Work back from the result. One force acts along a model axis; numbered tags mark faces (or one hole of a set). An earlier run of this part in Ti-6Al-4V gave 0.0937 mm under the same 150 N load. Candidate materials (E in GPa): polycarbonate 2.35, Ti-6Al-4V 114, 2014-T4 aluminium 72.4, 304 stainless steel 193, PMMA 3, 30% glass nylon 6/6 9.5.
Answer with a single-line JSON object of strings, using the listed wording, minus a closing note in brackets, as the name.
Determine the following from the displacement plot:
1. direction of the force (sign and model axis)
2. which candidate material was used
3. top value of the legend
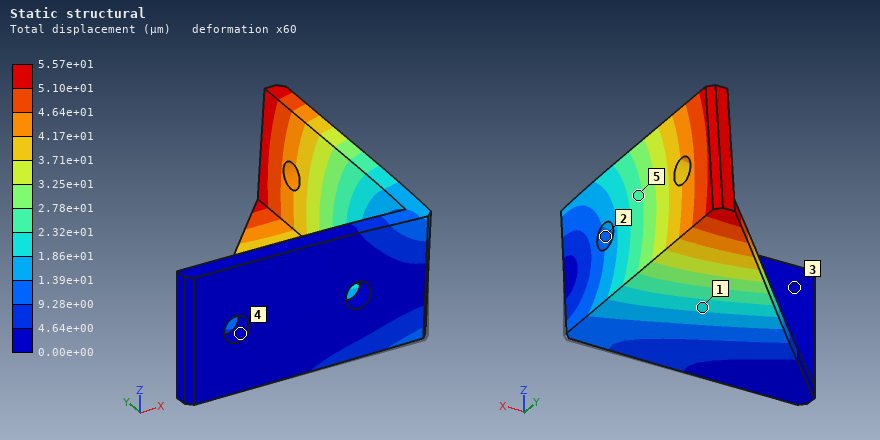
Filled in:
{"direction of the force": "+Z", "which candidate material was used": "304 stainless steel", "top value of the legend": "5.57e+01 µm"}
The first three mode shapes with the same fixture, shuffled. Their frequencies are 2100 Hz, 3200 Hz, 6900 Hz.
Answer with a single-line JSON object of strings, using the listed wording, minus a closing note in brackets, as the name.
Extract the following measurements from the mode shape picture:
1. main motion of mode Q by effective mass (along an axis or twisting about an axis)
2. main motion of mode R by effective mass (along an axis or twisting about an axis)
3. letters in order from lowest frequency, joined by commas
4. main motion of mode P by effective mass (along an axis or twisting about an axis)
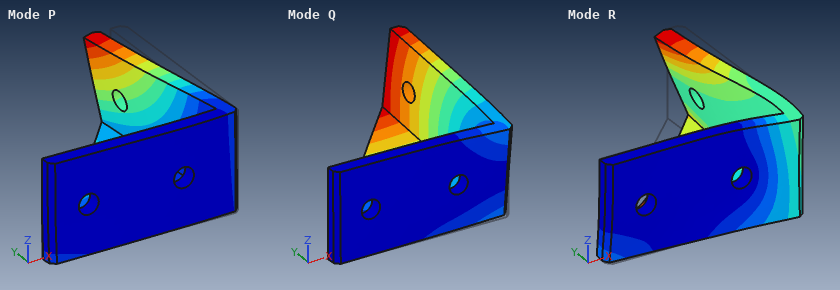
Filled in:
{"main motion of mode Q by effective mass": "along Z", "main motion of mode R by effective mass": "along Y", "letters in order from lowest frequency, joined by commas": "Q, P, R", "main motion of mode P by effective mass": "along X"}
